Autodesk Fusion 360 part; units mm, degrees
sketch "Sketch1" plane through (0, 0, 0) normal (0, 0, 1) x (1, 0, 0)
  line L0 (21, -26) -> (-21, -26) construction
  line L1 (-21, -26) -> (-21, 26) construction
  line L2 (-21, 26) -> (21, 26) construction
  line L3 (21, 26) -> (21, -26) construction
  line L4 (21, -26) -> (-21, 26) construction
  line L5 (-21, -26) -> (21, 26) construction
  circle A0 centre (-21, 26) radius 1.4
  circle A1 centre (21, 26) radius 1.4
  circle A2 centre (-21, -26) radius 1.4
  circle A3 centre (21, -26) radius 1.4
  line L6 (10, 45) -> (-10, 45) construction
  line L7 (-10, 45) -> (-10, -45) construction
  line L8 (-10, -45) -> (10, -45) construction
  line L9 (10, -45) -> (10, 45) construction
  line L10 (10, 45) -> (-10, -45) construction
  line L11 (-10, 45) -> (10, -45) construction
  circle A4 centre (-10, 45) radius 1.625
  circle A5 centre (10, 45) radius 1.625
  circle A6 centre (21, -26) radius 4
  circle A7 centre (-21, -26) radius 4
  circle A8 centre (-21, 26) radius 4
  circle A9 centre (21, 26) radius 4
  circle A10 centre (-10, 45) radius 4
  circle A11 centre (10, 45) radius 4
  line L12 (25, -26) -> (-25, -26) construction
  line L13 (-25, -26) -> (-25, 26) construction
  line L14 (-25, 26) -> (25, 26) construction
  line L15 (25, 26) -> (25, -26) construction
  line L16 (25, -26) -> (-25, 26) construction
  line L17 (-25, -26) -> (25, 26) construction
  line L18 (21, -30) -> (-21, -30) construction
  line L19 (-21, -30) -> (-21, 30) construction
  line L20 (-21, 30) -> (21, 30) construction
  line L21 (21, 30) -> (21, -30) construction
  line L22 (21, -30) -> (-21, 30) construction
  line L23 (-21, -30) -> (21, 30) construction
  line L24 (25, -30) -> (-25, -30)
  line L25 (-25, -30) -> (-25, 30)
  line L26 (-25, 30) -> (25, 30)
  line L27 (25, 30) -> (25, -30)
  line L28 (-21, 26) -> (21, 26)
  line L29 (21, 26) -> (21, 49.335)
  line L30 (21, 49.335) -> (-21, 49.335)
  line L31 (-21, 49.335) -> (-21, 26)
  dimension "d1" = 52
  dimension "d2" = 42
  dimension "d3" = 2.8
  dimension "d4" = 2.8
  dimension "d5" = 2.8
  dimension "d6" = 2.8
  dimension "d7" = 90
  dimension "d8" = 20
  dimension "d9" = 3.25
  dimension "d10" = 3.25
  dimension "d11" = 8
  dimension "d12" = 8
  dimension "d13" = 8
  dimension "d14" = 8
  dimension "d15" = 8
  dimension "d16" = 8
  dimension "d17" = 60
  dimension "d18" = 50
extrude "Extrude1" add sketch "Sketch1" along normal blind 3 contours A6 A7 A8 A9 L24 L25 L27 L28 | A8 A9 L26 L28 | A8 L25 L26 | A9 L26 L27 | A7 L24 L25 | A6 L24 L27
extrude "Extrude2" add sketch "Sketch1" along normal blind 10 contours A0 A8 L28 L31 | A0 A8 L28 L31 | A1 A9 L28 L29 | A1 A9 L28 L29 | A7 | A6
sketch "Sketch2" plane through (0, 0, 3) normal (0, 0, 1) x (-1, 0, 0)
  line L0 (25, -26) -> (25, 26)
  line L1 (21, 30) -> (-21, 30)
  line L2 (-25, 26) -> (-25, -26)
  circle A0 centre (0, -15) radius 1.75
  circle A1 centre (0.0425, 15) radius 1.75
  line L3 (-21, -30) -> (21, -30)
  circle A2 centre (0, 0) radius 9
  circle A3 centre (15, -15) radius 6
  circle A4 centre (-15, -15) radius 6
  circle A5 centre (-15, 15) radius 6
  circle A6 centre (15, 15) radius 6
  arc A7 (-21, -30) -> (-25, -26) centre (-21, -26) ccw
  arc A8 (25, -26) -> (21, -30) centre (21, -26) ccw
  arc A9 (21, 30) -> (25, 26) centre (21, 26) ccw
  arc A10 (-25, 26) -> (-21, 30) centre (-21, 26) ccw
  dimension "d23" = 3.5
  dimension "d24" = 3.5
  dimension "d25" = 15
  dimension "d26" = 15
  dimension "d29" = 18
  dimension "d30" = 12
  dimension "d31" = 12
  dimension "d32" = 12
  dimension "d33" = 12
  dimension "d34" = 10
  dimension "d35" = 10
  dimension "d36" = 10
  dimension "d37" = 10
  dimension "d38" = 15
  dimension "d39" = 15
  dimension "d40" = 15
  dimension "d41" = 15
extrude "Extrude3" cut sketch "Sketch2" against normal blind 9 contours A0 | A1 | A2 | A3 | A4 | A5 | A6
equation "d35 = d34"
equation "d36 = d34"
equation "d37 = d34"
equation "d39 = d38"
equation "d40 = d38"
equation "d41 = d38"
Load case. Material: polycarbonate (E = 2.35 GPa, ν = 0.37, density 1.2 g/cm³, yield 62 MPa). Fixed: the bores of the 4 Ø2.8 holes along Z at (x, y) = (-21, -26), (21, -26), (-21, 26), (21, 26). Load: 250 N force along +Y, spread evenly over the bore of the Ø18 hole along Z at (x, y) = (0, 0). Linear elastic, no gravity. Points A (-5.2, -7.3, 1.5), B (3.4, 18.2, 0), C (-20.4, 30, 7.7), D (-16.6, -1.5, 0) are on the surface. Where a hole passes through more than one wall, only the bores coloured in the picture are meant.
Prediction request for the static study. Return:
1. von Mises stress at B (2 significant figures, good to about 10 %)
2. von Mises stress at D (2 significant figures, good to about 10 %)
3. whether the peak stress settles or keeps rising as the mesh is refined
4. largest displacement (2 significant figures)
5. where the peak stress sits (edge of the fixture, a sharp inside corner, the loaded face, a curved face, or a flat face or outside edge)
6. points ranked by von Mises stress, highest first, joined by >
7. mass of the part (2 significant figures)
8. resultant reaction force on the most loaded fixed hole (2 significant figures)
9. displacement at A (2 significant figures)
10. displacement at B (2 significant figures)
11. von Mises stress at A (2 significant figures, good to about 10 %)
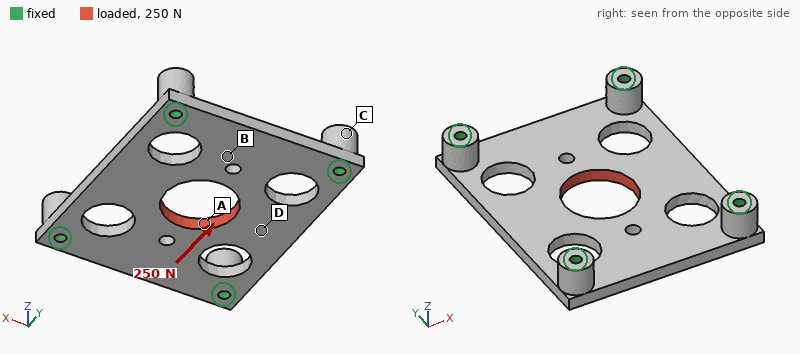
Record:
0.99 MPa
1.6 MPa
keeps rising
48 µm
edge of the fixture
A > D > B > C
9.6 g
67 N
45 µm
38 µm
2.2 MPa
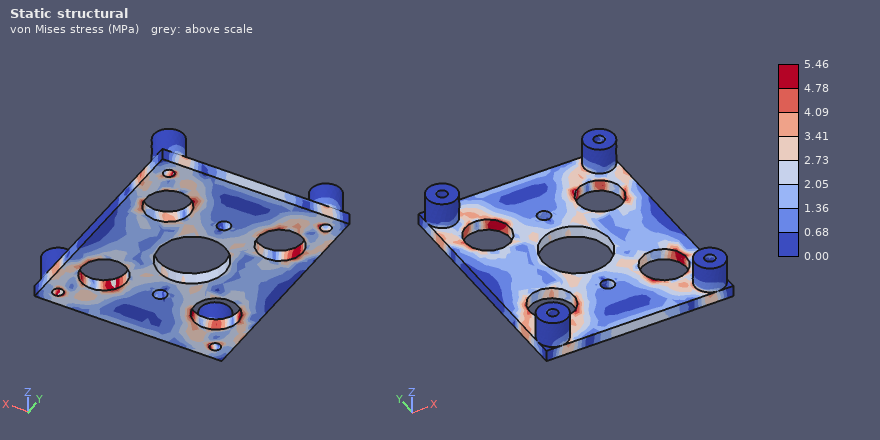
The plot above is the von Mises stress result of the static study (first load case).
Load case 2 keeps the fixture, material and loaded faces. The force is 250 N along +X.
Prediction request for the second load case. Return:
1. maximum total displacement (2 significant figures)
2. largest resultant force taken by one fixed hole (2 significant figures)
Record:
63 µm
70 N
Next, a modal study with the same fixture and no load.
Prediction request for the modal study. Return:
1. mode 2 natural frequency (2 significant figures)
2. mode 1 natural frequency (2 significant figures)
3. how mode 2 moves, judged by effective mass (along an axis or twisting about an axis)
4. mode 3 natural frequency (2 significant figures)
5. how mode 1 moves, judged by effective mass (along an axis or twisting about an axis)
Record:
1900 Hz
1300 Hz
twisting about Y
2400 Hz
along Z
